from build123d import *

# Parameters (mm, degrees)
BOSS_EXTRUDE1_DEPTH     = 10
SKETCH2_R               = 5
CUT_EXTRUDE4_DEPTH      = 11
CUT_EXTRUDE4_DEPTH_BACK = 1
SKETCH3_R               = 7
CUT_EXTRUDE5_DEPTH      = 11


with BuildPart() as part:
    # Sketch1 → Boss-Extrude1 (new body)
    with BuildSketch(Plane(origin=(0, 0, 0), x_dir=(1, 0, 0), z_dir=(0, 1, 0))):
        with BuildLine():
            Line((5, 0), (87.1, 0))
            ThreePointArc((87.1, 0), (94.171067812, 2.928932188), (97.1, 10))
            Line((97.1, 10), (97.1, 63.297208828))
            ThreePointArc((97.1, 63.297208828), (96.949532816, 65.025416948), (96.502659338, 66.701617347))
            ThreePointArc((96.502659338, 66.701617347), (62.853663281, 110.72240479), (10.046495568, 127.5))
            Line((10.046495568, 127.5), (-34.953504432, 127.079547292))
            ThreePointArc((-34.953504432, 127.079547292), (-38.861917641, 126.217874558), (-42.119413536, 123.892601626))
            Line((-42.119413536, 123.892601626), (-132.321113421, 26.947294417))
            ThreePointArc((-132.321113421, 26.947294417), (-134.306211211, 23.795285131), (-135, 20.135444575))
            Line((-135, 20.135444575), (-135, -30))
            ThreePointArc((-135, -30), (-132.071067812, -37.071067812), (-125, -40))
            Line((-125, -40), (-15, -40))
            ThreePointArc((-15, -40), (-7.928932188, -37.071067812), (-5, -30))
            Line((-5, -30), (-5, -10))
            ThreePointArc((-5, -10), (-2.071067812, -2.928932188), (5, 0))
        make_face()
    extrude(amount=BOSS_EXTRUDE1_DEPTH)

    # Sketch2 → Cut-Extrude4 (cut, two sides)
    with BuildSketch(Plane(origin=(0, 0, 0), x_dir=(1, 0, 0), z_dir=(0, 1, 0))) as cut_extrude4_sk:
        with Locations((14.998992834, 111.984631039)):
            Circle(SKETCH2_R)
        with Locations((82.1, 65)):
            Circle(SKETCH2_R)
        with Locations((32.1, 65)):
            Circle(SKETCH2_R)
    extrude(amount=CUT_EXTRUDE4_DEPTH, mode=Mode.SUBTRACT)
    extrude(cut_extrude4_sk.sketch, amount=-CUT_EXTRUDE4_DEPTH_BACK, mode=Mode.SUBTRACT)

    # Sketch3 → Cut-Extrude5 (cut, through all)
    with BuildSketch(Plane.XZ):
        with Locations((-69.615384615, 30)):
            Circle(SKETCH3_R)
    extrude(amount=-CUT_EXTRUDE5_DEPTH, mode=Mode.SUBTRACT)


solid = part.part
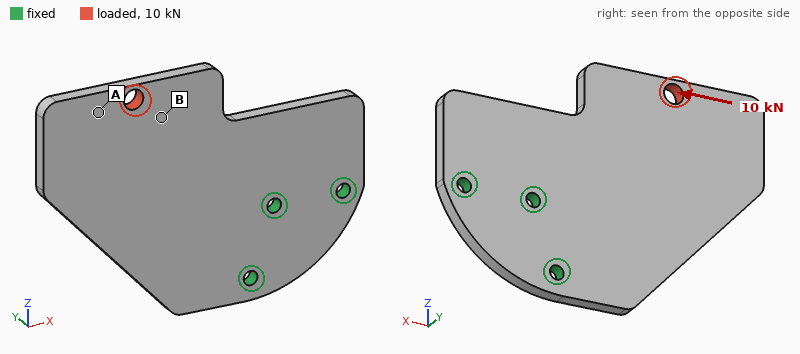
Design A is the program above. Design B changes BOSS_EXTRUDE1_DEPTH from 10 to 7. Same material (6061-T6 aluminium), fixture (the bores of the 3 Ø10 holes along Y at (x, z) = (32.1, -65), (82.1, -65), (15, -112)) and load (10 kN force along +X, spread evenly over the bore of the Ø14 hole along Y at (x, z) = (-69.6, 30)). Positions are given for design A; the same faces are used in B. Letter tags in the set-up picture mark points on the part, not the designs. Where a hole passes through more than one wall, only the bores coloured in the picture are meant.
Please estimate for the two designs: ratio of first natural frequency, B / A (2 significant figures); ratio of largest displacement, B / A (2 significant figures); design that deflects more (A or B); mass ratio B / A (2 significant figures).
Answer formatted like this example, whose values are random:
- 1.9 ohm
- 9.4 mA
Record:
- 0.71
- 1.4
- B
- 0.70
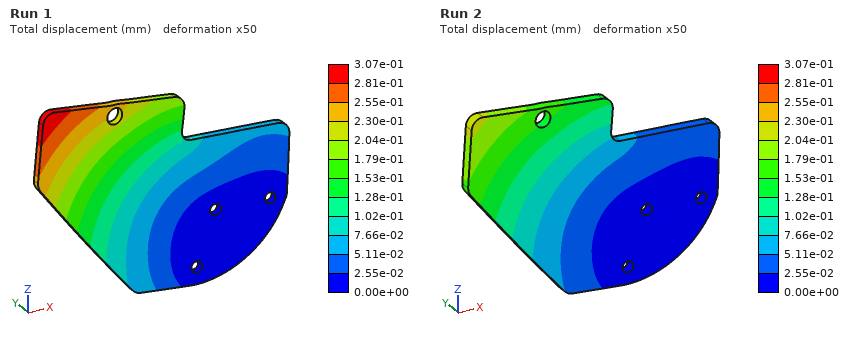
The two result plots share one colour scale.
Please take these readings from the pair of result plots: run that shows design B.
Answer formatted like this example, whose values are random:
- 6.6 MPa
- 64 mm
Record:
- Run 1
